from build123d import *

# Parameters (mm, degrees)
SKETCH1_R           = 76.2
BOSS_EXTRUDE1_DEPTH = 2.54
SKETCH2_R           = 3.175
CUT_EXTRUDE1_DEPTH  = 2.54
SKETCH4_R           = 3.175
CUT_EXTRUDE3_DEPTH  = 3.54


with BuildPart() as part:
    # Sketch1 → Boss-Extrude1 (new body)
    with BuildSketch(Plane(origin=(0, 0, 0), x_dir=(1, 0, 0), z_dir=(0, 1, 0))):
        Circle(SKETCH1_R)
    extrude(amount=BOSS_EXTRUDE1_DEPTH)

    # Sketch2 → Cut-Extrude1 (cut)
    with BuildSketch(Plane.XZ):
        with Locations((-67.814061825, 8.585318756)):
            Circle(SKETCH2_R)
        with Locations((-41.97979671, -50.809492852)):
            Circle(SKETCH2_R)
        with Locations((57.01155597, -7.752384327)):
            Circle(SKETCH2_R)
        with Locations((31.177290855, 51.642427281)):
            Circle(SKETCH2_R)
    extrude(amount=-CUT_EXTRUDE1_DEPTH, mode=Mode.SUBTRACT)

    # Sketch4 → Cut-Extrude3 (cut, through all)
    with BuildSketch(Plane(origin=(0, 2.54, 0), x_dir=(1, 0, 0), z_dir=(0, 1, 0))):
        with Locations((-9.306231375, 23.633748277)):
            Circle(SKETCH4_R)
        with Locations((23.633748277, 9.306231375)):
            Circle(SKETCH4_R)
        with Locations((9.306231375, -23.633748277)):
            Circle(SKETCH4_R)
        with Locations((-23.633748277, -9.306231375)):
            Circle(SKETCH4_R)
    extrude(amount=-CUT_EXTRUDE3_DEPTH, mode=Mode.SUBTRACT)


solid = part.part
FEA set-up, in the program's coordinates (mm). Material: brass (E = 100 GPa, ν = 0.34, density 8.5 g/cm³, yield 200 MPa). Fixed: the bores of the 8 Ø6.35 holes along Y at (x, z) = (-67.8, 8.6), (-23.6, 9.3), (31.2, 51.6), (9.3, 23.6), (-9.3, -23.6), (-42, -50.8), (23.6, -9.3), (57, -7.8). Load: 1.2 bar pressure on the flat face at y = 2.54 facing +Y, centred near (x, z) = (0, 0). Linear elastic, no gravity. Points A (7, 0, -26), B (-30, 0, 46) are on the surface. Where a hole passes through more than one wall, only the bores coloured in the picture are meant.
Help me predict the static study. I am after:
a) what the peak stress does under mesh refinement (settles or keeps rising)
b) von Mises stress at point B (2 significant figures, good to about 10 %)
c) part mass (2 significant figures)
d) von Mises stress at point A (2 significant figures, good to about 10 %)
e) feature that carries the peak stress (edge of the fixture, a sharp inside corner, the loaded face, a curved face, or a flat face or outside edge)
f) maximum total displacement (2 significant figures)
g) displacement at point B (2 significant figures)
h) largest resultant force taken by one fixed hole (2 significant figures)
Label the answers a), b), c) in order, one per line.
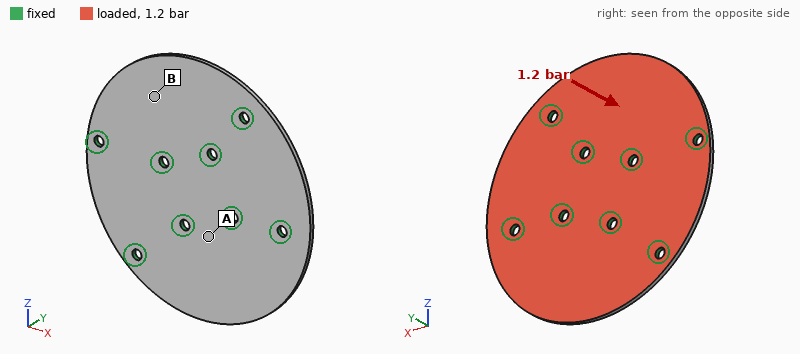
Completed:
a) keeps rising
b) 23 MPa
c) 390 g
d) 59 MPa
e) edge of the fixture
f) 0.61 mm
g) 0.27 mm
h) 330 N
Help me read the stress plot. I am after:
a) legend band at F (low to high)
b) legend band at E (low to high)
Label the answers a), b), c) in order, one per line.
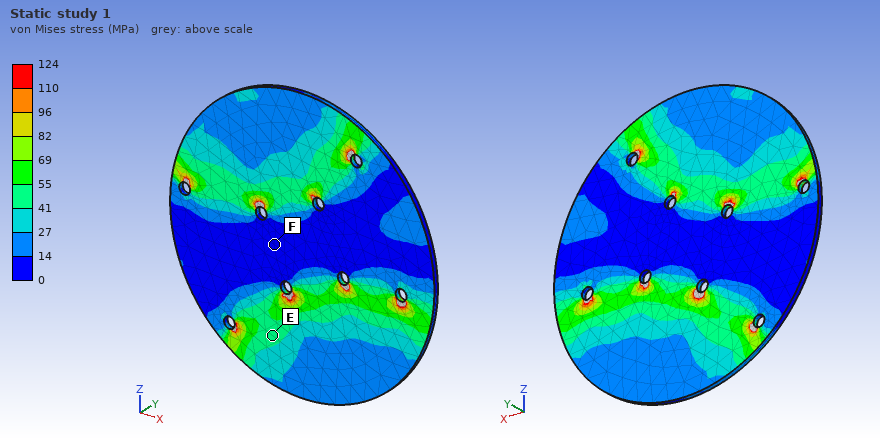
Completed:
a) 0 to 14 MPa
b) 41 to 55 MPa
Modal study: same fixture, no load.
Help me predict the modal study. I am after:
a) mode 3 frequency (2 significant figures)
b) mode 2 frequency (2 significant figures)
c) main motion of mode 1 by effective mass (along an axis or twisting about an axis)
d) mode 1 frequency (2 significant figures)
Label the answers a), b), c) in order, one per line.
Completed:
a) 1400 Hz
b) 700 Hz
c) along Y
d) 650 Hz
